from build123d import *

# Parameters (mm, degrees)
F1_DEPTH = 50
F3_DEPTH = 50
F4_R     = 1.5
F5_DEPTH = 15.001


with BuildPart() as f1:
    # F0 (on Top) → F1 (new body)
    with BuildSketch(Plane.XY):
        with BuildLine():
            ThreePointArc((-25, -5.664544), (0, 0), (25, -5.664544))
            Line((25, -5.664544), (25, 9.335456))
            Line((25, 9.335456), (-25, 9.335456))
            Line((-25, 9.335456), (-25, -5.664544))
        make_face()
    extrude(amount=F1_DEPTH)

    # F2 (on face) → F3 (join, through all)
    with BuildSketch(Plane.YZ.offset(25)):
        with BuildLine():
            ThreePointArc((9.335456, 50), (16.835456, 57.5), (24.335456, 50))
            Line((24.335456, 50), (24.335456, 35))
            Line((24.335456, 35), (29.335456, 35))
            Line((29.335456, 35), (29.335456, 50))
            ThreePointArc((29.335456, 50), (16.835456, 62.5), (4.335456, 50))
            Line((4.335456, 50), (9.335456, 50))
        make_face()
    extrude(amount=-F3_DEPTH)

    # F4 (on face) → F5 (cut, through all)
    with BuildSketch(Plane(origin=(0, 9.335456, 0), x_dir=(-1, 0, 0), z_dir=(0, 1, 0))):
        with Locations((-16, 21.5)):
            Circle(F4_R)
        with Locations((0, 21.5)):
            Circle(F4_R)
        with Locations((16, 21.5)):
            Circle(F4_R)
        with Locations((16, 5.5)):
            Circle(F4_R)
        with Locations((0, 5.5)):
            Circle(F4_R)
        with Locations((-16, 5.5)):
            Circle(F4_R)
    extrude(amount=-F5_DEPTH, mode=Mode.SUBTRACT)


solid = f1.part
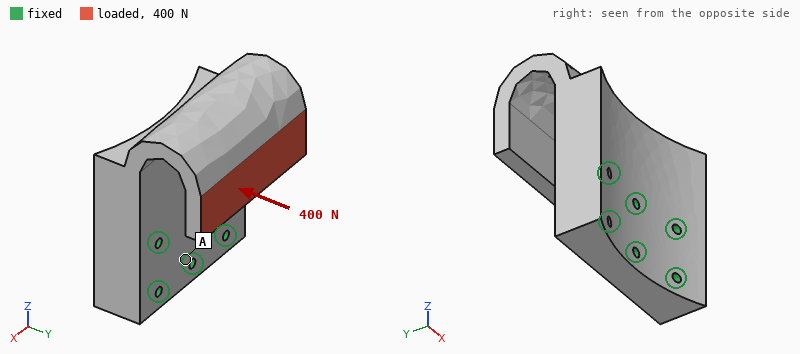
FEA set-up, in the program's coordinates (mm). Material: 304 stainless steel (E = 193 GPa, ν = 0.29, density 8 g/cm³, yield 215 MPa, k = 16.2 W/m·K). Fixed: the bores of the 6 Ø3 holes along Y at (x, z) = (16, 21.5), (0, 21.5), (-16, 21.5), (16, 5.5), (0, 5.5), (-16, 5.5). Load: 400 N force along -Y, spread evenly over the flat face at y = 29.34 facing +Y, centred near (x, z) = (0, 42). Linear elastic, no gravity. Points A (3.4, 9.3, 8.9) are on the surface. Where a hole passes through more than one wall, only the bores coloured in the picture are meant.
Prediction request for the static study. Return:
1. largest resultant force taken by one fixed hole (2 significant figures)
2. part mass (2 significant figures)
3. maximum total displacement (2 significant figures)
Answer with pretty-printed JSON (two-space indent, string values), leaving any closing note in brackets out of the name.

{
  "largest resultant force taken by one fixed hole": "210 N",
  "part mass": "310 g",
  "maximum total displacement": "42 µm"
}
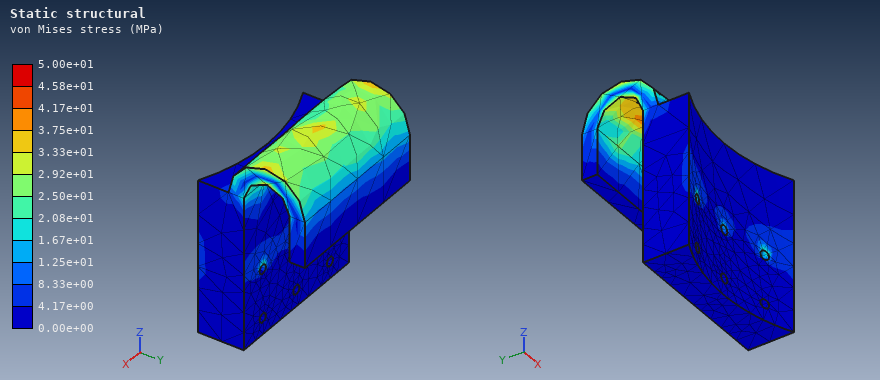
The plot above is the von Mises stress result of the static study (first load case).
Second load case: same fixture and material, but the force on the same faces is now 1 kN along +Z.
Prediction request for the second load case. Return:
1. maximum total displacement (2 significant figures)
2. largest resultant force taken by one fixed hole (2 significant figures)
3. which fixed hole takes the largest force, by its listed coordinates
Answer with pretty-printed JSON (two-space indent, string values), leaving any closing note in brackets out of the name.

{
  "maximum total displacement": "0.12 mm",
  "largest resultant force taken by one fixed hole": "610 N",
  "which fixed hole takes the largest force, by its listed coordinates": "(0, 21.5)"
}
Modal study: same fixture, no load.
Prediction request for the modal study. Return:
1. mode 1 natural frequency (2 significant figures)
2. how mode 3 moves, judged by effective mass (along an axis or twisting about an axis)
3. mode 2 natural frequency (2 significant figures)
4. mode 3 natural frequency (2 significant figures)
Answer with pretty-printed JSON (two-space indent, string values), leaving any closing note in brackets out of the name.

{
  "mode 1 natural frequency": "2300 Hz",
  "how mode 3 moves, judged by effective mass": "along Y",
  "mode 2 natural frequency": "3200 Hz",
  "mode 3 natural frequency": "3600 Hz"
}
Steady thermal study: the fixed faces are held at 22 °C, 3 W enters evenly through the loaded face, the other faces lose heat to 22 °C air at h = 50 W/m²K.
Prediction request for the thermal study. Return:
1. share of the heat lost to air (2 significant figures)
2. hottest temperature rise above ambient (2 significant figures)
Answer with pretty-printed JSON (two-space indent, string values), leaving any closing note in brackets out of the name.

{
  "share of the heat lost to air": "79 %",
  "hottest temperature rise above ambient": "17 K"
}
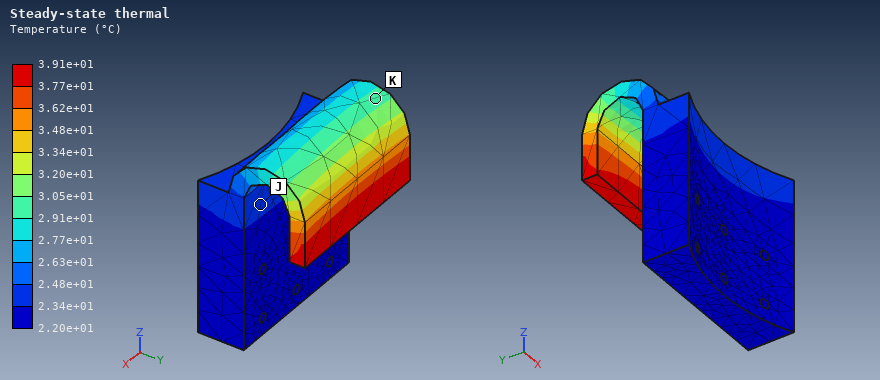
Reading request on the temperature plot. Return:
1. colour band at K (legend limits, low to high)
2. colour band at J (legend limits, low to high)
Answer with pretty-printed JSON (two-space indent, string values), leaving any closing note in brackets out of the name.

{
  "colour band at K": "2.91e+01 to 3.05e+01 °C",
  "colour band at J": "2.34e+01 to 2.48e+01 °C"
}
